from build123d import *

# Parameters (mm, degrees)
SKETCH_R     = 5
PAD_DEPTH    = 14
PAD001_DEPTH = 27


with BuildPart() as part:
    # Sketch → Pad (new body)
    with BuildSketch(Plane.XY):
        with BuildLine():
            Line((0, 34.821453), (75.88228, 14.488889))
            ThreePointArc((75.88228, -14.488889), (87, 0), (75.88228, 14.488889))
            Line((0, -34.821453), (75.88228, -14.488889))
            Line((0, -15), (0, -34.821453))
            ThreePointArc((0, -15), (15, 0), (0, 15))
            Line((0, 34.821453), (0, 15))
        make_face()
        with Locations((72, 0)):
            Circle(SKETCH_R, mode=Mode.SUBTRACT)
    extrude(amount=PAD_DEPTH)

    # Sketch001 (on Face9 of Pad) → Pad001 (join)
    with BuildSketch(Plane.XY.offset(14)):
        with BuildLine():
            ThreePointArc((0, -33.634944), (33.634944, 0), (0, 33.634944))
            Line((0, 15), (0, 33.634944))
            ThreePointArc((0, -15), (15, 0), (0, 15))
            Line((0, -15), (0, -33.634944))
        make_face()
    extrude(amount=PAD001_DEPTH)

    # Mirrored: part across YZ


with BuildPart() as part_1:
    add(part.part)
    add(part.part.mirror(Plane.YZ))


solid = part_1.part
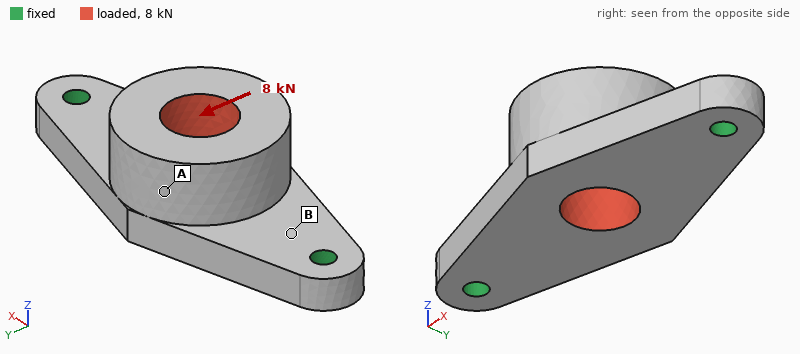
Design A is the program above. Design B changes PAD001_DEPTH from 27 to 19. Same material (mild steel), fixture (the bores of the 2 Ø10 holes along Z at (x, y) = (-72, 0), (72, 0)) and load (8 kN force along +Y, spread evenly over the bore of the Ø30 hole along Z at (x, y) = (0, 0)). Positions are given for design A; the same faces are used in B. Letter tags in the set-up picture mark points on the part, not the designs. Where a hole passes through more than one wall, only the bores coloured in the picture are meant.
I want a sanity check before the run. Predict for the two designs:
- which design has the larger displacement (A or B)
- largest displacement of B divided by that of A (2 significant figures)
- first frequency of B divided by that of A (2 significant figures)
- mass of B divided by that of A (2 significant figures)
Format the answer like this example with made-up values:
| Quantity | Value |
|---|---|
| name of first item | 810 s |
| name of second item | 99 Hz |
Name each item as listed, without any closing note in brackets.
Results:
| Quantity | Value |
|---|---|
| which design has the larger displacement | A |
| largest displacement of B divided by that of A | 0.68 |
| first frequency of B divided by that of A | 1.2 |
| mass of B divided by that of A | 0.87 |
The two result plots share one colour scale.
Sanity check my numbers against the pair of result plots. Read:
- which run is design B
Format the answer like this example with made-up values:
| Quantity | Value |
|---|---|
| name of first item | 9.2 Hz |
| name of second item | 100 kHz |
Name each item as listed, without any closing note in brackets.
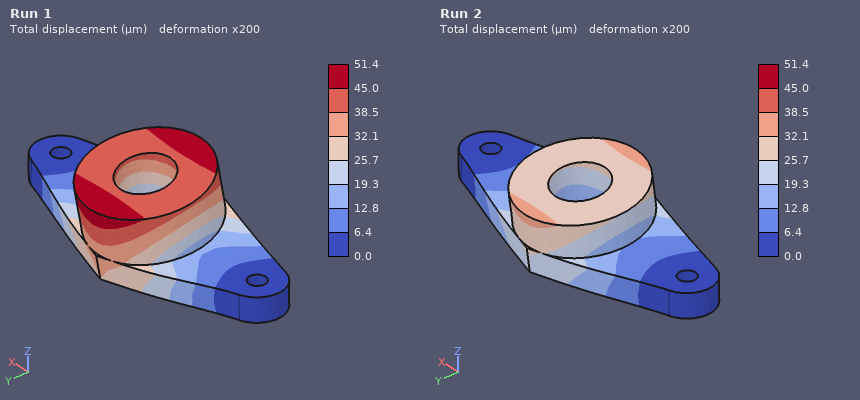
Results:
| Quantity | Value |
|---|---|
| which run is design B | Run 2 |
